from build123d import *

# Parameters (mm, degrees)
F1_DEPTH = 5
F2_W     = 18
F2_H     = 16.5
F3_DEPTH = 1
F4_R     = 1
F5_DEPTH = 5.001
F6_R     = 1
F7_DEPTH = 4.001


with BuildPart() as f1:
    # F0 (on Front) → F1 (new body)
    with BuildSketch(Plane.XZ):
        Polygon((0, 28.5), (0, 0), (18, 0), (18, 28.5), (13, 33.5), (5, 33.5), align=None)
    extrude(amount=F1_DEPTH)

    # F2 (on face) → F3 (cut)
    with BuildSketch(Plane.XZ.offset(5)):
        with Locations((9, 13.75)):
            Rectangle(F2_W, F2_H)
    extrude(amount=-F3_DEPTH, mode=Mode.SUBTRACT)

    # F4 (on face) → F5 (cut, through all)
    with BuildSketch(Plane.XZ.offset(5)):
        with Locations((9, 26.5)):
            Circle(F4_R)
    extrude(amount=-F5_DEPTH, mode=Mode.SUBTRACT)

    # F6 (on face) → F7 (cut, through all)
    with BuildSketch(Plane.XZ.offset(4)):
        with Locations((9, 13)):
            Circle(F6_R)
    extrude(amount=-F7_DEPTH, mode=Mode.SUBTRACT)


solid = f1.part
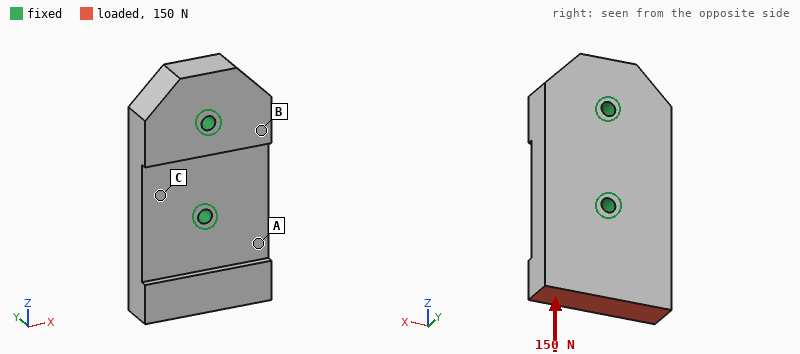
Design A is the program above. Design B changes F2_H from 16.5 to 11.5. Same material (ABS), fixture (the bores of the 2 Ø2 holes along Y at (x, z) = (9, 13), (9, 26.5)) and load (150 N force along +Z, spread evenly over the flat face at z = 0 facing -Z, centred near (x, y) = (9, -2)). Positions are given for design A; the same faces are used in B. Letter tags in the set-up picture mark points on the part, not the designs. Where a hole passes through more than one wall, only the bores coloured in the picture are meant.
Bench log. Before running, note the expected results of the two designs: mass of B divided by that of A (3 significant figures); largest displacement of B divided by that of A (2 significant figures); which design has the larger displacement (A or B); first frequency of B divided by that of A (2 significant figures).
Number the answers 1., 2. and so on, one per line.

1. 1.04
2. 0.87
3. A
4. 1.00
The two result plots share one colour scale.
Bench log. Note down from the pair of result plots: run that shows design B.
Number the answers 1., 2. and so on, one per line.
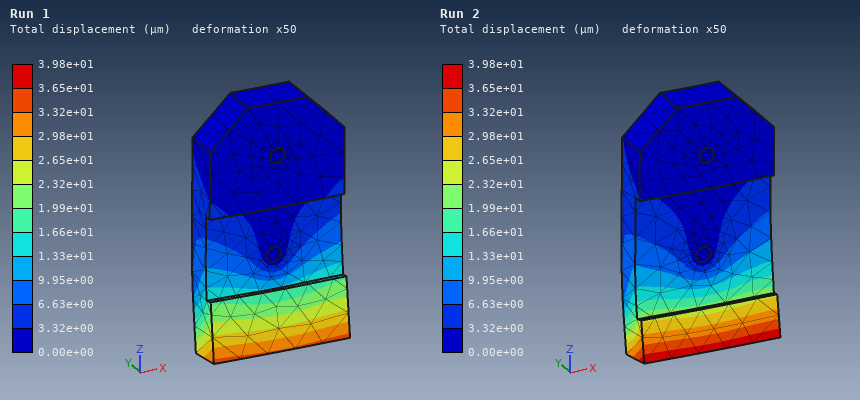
1. Run 1
